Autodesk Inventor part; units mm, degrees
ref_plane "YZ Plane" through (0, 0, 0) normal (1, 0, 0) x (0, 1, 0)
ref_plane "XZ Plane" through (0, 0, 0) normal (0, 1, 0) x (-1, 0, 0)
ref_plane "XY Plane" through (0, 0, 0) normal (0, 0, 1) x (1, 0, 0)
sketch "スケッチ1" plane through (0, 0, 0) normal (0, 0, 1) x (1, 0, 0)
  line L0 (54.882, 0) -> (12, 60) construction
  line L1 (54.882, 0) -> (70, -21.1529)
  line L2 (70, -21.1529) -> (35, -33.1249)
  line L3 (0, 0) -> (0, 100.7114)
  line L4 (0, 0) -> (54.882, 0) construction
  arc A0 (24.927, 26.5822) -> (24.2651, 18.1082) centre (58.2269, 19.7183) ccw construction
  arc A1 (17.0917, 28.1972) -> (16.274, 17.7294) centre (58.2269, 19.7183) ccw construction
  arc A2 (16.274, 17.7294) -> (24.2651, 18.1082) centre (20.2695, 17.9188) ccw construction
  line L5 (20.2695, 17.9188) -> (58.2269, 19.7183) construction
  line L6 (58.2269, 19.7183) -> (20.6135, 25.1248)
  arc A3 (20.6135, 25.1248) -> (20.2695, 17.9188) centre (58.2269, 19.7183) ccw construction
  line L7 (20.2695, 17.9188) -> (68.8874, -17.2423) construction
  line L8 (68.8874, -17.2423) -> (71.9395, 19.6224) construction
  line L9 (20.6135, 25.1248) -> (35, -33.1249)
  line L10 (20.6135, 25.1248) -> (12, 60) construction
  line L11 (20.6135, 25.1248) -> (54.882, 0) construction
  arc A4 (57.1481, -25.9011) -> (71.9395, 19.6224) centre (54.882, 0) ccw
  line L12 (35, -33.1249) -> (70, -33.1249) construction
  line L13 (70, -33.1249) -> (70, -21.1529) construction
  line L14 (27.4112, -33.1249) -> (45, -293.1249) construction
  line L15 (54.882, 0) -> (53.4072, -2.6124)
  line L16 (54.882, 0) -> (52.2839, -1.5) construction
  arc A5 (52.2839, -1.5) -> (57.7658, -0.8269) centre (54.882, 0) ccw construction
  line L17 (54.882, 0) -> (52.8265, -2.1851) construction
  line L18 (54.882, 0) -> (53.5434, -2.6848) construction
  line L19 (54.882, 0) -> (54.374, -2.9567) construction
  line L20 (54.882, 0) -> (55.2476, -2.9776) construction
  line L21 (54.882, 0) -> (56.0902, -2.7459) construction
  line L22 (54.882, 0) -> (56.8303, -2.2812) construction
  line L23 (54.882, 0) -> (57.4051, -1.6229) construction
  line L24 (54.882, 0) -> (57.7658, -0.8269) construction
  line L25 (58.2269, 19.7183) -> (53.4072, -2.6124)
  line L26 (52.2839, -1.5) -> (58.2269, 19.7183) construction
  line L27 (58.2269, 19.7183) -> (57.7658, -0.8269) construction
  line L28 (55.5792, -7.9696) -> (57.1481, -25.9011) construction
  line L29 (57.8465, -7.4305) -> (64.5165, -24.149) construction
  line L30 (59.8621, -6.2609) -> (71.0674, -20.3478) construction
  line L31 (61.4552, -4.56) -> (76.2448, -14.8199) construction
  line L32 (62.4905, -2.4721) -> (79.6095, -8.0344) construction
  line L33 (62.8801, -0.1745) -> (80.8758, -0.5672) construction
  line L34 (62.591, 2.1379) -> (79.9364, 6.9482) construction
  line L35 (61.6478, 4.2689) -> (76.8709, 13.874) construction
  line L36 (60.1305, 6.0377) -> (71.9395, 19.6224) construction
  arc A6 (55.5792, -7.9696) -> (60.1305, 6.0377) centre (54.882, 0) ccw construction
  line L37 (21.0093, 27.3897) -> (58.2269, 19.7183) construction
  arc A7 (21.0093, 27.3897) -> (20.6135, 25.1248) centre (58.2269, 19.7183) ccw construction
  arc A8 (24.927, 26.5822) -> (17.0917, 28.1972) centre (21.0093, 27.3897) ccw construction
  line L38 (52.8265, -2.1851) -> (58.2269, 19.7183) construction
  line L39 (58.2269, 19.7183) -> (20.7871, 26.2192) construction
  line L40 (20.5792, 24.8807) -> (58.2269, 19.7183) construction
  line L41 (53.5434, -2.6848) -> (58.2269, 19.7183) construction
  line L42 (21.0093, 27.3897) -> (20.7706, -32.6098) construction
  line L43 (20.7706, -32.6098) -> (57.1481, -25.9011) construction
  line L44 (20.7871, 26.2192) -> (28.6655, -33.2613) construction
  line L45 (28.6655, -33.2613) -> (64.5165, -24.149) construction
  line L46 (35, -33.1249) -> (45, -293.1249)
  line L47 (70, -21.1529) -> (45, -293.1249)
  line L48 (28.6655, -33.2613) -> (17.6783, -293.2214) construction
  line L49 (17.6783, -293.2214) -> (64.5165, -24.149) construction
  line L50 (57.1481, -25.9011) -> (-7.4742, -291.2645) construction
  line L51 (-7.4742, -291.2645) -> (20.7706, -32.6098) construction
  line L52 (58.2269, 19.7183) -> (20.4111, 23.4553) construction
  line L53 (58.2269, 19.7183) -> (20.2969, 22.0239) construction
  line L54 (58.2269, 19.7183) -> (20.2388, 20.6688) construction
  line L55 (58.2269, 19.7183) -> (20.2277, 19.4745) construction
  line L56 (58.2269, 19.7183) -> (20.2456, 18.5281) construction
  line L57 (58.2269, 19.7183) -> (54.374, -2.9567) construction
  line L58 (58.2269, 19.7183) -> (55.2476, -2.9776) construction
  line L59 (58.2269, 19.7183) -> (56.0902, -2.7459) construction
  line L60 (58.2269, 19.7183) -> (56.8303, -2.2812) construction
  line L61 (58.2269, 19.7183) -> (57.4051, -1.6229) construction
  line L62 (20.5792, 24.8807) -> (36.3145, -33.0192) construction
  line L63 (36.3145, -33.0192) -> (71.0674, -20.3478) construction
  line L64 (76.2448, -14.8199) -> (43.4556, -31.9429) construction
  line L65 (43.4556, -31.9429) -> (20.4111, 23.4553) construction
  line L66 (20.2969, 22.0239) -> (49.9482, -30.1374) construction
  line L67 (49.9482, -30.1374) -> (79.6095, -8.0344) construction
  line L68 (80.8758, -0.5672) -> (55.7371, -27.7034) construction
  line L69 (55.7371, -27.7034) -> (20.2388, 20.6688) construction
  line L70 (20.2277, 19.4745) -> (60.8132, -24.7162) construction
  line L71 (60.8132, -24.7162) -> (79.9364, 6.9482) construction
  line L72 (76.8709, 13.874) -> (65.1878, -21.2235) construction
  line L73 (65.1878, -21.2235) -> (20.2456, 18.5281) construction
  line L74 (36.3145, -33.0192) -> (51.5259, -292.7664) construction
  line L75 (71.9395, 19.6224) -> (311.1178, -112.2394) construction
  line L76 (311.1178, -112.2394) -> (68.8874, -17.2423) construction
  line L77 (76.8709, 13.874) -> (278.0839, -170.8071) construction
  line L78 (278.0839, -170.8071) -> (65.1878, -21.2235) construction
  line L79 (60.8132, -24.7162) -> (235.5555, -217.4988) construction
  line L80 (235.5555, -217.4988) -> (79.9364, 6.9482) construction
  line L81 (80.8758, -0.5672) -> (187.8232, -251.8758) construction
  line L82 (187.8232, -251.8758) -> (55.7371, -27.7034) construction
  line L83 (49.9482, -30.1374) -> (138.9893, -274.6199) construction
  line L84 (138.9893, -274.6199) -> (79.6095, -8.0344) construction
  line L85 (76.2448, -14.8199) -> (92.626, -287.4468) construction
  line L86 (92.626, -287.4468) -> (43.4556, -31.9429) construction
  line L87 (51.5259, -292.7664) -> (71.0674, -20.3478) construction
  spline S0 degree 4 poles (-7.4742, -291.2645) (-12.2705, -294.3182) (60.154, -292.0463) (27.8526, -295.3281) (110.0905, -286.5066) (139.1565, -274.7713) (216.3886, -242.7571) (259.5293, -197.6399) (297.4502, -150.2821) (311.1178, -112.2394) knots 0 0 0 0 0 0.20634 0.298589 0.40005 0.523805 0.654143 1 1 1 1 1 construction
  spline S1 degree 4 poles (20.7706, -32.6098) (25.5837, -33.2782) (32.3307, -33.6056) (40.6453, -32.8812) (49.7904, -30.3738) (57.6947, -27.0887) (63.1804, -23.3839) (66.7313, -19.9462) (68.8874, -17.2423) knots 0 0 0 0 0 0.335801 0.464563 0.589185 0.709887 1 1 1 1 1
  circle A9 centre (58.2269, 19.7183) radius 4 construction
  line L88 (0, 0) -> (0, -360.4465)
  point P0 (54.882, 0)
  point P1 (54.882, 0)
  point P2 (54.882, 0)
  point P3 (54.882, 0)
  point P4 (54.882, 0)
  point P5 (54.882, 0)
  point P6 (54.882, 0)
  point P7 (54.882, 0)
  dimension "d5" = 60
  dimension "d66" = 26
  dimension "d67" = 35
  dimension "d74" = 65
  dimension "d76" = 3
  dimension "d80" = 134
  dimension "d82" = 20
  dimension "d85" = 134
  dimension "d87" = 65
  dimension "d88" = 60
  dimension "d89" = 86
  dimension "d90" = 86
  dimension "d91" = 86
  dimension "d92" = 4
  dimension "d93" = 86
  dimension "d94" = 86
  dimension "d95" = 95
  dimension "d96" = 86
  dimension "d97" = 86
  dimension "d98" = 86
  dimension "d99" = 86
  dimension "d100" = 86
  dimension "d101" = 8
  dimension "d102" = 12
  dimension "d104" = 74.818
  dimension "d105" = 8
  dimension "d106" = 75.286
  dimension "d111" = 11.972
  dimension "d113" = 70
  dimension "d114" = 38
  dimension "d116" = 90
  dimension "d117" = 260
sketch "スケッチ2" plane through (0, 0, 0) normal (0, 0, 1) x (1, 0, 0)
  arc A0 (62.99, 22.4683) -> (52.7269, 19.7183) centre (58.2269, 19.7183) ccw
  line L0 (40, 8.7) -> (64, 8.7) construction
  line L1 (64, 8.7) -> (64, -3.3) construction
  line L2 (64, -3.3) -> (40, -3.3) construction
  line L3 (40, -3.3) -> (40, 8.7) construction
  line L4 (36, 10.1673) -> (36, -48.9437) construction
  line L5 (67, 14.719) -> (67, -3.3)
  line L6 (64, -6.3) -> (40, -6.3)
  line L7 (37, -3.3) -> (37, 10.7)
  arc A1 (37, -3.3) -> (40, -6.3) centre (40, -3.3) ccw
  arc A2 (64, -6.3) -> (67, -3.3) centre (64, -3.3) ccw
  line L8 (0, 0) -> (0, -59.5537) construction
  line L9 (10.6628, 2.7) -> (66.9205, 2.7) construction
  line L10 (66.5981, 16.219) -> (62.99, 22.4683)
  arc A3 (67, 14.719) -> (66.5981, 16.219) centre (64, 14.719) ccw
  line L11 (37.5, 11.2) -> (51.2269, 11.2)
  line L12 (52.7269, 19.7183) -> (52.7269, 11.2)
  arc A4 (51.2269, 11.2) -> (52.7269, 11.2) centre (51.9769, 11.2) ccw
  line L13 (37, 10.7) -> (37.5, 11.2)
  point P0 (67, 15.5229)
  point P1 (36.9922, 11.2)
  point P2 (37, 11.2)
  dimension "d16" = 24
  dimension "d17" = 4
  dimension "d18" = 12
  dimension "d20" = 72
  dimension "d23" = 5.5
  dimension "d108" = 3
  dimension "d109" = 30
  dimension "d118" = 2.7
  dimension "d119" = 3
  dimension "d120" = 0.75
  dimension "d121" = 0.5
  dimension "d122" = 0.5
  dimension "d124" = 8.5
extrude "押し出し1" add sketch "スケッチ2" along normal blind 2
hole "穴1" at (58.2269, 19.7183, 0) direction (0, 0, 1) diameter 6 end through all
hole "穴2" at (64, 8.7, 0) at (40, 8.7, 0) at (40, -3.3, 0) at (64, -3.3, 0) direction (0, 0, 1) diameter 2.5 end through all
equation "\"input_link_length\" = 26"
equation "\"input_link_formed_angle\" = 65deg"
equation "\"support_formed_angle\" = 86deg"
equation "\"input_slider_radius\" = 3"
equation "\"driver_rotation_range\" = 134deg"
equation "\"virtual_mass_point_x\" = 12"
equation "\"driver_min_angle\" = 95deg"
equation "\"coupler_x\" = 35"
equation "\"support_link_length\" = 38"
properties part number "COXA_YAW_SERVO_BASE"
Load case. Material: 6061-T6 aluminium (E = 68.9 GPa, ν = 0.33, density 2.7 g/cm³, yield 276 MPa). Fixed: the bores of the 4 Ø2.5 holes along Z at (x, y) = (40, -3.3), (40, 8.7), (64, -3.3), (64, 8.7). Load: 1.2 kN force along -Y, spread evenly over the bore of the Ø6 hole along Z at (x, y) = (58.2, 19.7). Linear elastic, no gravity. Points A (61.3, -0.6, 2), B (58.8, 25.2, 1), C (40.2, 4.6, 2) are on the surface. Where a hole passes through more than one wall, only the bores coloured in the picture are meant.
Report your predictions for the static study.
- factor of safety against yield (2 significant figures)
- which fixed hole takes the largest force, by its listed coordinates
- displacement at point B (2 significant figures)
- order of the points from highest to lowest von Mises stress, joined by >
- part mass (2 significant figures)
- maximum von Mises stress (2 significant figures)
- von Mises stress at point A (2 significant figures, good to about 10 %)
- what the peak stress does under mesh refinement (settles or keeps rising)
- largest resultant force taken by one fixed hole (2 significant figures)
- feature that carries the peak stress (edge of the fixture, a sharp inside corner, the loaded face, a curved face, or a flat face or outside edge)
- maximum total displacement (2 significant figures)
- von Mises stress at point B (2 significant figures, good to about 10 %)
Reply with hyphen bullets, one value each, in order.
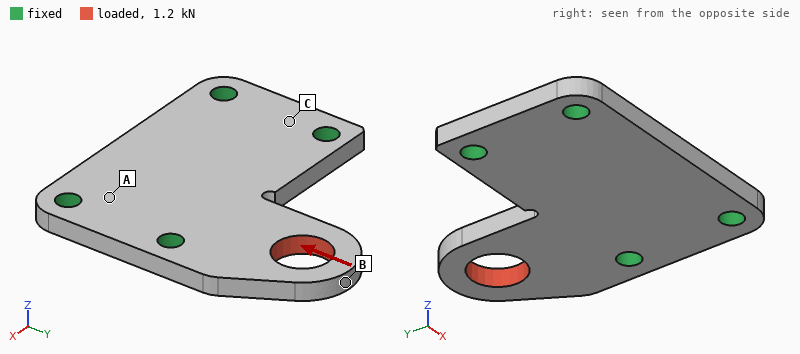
- 1.2
- (64, 8.7)
- 30 µm
- B > A > C
- 3.4 g
- 230 MPa
- 30 MPa
- settles
- 670 N
- a curved face
- 30 µm
- 78 MPa
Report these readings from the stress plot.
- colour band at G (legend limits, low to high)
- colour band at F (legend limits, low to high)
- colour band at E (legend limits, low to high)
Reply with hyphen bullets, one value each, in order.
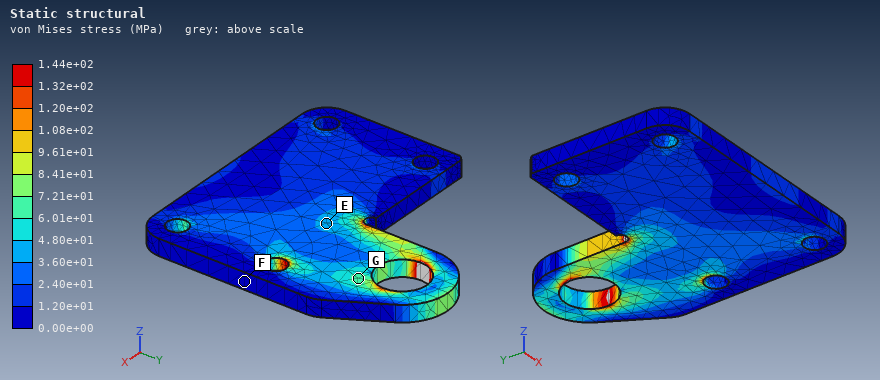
- 6.01e+01 to 7.21e+01 MPa
- 0.00e+00 to 1.20e+01 MPa
- 3.60e+01 to 4.80e+01 MPa
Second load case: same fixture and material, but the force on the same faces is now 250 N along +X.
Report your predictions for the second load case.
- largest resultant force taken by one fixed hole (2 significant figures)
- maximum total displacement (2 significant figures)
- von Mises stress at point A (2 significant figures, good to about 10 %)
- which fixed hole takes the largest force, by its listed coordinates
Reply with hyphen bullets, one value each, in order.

- 290 N
- 19 µm
- 8.4 MPa
- (64, 8.7)
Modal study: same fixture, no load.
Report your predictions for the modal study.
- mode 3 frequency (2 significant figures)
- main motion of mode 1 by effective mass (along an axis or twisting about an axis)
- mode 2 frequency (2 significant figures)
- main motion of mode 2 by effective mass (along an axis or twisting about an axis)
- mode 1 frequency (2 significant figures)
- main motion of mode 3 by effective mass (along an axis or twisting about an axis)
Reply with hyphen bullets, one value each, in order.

- 21 kHz
- along Z
- 17 kHz
- along Z
- 7500 Hz
- along Z
